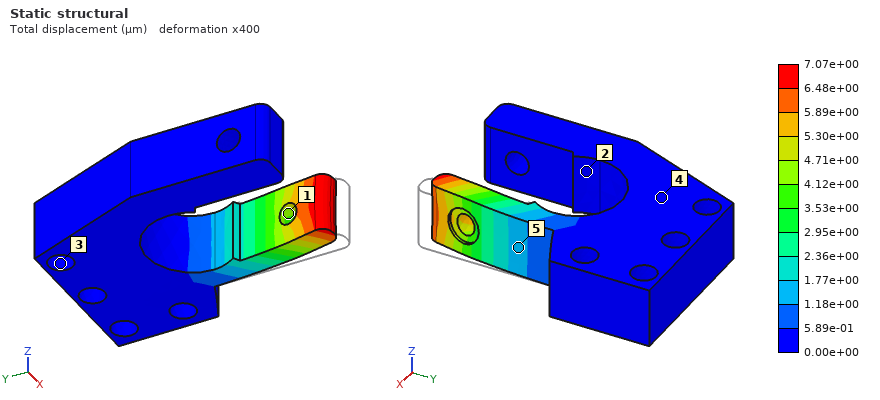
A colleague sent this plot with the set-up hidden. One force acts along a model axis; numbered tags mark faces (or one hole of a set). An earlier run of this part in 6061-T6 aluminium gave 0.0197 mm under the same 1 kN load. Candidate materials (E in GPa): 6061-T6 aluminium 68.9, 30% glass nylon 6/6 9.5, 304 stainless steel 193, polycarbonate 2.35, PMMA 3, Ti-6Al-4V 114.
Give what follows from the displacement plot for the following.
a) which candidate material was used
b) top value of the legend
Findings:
304 stainless steel
7.07e+00 µm
